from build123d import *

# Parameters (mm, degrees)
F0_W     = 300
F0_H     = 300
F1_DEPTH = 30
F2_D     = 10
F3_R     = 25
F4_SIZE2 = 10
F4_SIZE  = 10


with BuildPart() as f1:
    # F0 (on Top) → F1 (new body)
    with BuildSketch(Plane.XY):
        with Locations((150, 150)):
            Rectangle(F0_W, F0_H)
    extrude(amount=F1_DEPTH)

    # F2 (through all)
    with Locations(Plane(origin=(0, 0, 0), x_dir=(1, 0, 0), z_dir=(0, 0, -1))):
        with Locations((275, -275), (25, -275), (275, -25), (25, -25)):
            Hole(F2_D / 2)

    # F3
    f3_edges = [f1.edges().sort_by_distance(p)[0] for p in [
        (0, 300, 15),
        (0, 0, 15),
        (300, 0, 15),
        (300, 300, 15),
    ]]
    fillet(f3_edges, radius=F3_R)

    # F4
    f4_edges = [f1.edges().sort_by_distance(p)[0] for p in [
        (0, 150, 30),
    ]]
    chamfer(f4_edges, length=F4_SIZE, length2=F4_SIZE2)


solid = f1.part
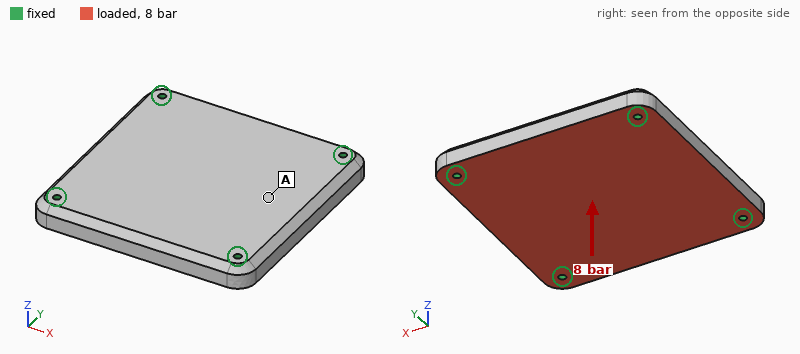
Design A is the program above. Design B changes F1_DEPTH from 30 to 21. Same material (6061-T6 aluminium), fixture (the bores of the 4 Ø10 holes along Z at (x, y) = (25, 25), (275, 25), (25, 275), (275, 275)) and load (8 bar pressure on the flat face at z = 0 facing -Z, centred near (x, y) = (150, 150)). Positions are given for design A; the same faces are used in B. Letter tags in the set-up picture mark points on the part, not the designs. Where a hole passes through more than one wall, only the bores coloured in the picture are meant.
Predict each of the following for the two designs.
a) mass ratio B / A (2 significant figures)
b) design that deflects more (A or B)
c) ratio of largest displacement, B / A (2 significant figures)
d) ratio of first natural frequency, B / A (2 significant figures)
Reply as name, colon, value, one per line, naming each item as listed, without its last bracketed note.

mass ratio B / A: 0.69
design that deflects more: B
ratio of largest displacement, B / A: 2.6
ratio of first natural frequency, B / A: 0.74
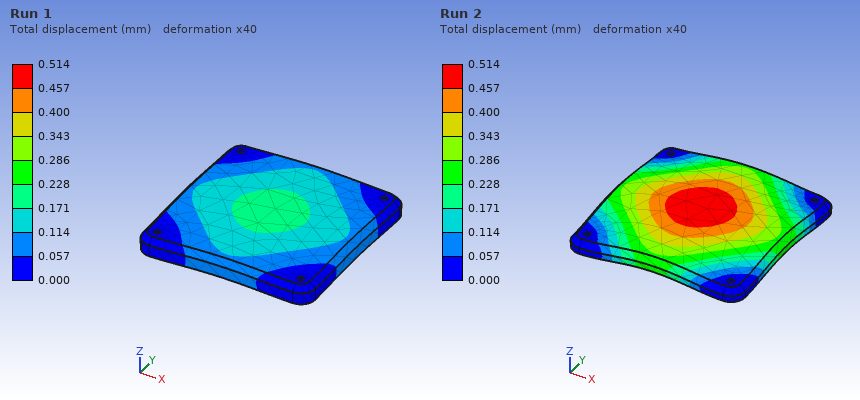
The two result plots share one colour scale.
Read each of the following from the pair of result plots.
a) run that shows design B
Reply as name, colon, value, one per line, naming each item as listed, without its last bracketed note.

run that shows design B: Run 2
